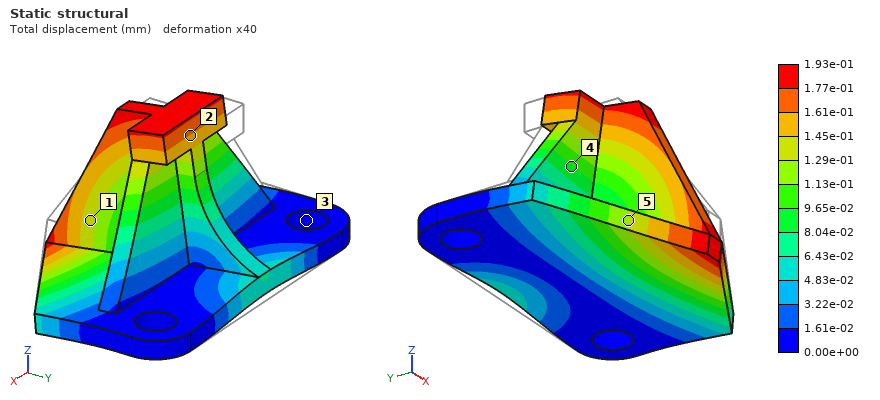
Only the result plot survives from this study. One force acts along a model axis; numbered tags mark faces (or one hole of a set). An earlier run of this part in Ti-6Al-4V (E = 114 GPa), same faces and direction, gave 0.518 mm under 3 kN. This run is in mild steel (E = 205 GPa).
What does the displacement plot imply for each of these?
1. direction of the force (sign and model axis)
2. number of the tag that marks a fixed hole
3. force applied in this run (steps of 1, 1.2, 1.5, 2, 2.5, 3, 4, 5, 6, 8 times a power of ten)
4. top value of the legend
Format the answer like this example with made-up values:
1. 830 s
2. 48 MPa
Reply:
1. -Y
2. 3
3. 2 kN
4. 1.93e-01 mm
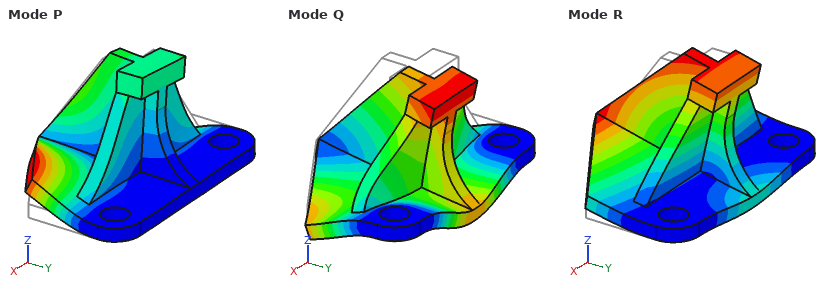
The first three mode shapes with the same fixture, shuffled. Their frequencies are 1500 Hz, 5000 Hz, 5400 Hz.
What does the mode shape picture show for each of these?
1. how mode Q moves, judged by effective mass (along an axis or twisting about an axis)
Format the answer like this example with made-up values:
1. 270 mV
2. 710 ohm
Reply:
1. along Z
